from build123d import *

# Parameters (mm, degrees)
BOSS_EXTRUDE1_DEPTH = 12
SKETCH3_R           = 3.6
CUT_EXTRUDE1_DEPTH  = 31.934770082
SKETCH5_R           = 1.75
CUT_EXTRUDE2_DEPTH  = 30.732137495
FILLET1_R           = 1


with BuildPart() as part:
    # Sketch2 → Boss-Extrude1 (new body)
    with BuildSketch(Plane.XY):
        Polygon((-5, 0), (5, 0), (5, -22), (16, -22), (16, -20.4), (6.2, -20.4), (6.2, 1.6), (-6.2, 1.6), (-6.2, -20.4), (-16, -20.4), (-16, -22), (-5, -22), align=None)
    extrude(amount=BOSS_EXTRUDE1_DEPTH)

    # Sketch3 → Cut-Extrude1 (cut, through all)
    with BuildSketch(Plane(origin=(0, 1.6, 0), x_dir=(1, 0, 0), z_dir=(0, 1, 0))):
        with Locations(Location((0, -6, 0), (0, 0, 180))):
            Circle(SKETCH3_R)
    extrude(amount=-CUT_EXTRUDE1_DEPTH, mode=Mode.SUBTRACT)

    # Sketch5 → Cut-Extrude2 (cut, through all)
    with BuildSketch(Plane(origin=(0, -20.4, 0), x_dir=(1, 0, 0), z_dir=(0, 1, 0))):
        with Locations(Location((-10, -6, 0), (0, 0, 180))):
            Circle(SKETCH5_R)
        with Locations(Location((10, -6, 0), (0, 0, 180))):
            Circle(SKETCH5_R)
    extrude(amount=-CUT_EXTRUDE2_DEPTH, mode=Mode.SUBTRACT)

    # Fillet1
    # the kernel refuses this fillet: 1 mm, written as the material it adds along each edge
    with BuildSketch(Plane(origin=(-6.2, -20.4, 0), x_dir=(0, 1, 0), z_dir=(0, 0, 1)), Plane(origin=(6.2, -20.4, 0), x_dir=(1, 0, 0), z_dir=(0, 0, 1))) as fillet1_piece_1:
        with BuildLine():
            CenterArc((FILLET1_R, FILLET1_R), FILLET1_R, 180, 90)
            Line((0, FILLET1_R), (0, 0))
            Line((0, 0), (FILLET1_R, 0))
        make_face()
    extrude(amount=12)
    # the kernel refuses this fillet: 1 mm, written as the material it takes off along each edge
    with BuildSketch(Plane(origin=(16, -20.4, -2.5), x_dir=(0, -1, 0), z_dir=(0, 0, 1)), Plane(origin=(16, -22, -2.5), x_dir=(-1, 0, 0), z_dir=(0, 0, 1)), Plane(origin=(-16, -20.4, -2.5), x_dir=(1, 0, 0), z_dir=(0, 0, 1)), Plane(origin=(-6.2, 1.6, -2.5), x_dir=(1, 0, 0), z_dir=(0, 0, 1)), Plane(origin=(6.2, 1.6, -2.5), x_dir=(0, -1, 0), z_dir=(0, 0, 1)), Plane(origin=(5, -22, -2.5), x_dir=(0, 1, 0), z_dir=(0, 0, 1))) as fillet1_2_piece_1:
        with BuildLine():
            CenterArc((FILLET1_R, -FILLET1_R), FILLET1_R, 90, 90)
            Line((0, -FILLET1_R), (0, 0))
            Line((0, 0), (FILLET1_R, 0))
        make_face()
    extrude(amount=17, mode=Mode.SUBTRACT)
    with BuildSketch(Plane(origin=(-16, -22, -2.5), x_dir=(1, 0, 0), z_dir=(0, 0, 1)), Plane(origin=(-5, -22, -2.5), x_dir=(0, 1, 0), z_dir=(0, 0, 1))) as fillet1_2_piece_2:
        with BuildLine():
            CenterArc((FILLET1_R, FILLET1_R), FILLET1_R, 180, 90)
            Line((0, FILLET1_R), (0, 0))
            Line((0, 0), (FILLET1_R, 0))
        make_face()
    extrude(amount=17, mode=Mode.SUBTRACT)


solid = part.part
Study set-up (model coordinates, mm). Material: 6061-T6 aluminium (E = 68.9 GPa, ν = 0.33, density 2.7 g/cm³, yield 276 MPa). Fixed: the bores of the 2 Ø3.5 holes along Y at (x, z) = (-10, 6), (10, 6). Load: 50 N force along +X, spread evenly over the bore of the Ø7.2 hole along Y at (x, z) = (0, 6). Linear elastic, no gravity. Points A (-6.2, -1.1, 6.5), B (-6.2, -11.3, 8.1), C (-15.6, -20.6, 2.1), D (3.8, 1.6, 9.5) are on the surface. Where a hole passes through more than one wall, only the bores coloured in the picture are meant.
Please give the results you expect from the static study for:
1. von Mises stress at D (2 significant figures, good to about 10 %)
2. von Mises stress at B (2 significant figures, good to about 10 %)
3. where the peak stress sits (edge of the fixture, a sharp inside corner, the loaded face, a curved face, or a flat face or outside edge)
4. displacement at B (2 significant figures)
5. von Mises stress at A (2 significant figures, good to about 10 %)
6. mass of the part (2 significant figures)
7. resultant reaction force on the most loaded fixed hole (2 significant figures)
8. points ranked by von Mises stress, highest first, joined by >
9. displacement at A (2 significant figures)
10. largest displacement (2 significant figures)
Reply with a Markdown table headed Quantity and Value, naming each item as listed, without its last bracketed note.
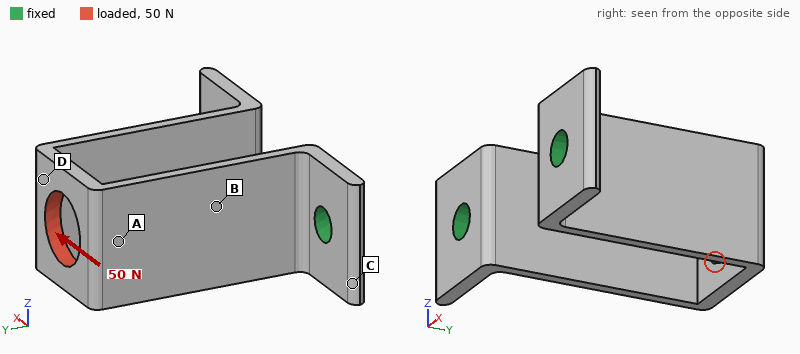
| Quantity | Value |
|---|---|
| von Mises stress at D | 47 MPa |
| von Mises stress at B | 15 MPa |
| where the peak stress sits | a curved face |
| displacement at B | 0.080 mm |
| von Mises stress at A | 64 MPa |
| mass of the part | 3.1 g |
| resultant reaction force on the most loaded fixed hole | 54 N |
| points ranked by von Mises stress, highest first, joined by > | A > D > B > C |
| displacement at A | 0.19 mm |
| largest displacement | 0.19 mm |
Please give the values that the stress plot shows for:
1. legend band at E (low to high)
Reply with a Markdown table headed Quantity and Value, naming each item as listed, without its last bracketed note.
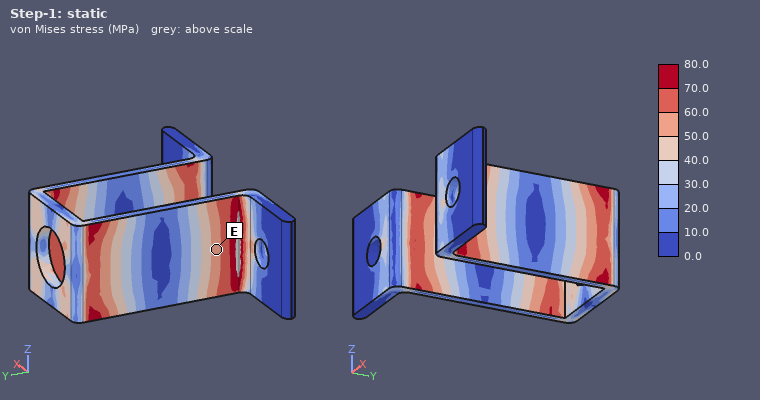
| Quantity | Value |
|---|---|
| legend band at E | 50.0 to 60.0 MPa |
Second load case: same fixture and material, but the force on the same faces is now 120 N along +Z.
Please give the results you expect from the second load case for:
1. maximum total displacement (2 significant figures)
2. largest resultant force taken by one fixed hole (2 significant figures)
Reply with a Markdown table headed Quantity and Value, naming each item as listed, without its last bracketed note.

| Quantity | Value |
|---|---|
| maximum total displacement | 0.19 mm |
| largest resultant force taken by one fixed hole | 60 N |
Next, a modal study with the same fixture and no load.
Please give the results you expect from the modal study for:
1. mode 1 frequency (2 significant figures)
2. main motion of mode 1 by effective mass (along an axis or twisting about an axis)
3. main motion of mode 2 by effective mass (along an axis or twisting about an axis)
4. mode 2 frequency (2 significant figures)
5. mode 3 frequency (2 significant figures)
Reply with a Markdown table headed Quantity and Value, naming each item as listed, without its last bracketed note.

| Quantity | Value |
|---|---|
| mode 1 frequency | 2500 Hz |
| main motion of mode 1 by effective mass | along X |
| main motion of mode 2 by effective mass | along Z |
| mode 2 frequency | 4100 Hz |
| mode 3 frequency | 5400 Hz |
